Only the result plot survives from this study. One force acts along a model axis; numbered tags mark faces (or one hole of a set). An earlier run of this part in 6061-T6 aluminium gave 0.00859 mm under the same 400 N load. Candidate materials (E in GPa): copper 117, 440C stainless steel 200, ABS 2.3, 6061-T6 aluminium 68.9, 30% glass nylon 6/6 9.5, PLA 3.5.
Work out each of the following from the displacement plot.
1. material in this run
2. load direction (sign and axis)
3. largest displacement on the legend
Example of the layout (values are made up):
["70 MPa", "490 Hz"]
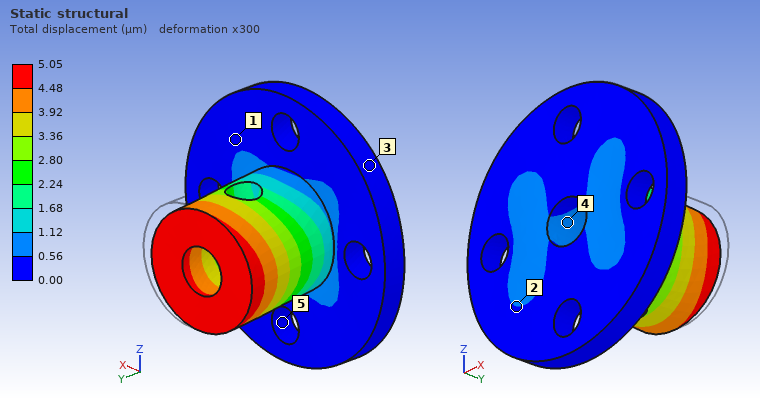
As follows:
["copper", "-X", "5.05 µm"]
